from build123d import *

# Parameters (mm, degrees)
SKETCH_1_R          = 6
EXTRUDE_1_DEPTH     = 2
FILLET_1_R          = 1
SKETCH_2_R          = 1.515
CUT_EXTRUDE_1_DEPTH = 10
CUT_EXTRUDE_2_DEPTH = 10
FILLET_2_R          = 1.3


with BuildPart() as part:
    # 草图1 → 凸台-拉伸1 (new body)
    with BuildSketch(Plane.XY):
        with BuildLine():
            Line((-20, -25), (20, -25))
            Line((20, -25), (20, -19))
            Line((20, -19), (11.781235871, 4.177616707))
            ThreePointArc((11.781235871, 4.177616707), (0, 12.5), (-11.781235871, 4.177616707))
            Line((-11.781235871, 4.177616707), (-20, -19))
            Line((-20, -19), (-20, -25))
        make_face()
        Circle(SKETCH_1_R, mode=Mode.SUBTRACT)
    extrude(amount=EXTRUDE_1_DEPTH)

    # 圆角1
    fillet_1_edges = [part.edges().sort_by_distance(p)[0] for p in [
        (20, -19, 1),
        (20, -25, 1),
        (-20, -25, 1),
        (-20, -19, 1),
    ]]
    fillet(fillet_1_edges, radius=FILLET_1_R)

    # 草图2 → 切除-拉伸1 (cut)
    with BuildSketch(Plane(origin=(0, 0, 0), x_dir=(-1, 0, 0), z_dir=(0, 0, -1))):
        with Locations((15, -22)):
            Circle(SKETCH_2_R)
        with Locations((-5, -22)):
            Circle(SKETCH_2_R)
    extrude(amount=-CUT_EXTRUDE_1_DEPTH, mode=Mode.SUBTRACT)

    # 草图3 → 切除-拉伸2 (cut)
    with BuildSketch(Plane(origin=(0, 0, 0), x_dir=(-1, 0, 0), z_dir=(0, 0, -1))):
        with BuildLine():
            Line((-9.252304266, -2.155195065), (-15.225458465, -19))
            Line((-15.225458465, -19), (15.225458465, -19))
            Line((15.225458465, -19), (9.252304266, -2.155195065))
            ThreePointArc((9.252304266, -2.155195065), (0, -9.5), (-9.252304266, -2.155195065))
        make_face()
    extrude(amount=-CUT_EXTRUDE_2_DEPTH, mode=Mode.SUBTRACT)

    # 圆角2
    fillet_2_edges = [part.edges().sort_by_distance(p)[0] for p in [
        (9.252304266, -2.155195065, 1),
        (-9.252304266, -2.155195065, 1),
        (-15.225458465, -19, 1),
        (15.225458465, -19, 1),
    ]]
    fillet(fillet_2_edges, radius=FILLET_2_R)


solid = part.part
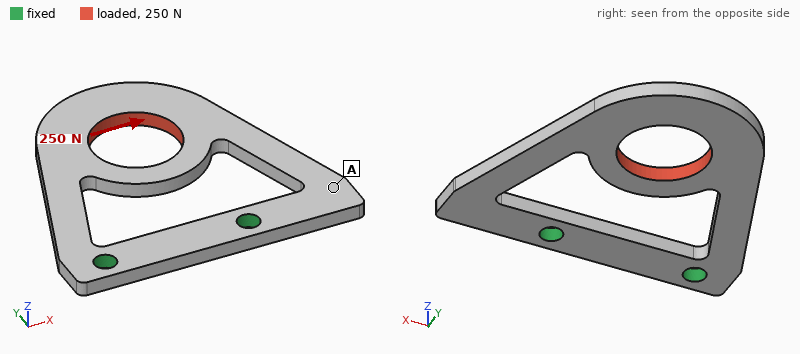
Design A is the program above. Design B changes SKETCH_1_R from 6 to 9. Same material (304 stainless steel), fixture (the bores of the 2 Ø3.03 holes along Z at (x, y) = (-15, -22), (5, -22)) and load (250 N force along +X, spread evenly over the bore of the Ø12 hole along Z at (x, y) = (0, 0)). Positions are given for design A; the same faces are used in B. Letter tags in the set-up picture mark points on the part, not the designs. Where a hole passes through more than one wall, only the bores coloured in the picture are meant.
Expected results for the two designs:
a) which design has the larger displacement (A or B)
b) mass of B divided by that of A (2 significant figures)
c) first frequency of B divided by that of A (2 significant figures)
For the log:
B
0.79
1.2
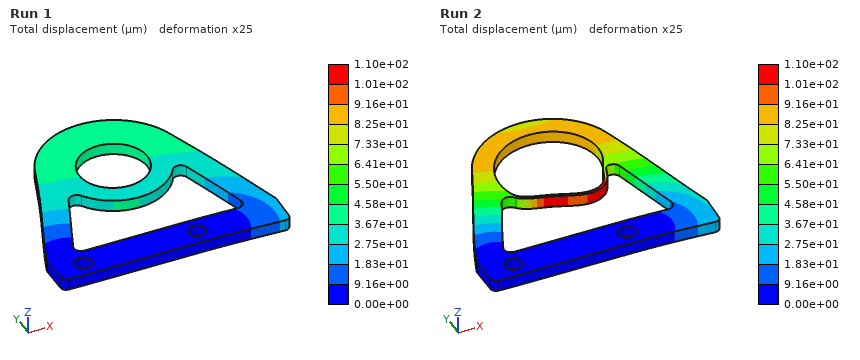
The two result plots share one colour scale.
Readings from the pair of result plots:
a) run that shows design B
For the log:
Run 2
